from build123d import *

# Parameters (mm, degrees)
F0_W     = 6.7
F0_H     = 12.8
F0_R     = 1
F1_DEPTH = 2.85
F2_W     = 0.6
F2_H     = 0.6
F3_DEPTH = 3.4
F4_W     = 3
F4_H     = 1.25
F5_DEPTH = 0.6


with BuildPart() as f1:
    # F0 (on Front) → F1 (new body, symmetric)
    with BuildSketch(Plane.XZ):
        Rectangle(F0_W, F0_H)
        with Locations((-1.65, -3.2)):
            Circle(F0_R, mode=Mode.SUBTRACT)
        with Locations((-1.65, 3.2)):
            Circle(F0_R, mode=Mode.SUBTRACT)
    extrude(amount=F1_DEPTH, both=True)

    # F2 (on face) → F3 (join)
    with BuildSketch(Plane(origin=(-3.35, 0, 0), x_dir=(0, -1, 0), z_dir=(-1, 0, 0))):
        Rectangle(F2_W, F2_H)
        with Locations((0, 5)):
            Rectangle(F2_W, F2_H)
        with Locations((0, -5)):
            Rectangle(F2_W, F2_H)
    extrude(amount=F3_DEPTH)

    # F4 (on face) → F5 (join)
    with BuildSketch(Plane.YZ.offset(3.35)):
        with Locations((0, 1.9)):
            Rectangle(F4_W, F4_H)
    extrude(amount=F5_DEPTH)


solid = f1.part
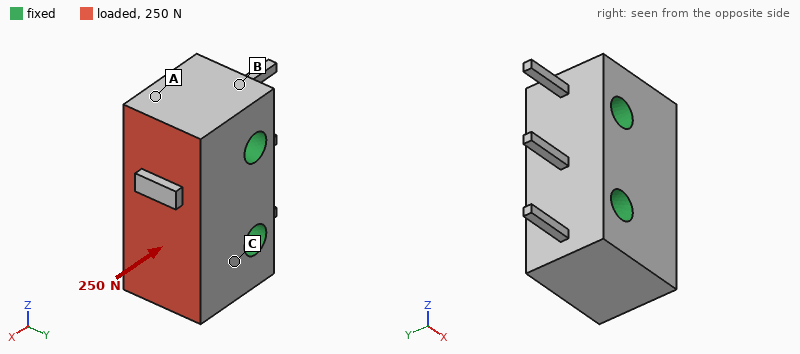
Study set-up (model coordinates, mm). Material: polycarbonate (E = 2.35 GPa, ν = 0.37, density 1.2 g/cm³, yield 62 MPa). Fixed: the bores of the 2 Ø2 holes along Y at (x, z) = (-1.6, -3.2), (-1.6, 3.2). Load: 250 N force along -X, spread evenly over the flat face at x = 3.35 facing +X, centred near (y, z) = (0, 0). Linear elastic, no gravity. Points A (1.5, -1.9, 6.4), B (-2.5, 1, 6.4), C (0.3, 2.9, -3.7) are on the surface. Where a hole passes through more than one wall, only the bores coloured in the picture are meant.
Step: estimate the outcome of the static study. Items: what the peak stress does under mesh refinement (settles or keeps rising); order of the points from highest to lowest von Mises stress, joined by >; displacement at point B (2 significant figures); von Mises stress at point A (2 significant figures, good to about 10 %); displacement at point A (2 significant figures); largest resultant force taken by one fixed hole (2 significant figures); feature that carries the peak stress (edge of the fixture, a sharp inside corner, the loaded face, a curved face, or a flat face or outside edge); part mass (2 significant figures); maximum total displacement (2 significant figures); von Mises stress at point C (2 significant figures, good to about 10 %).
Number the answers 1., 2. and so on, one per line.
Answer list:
1. keeps rising
2. C > A > B
3. 5.3 µm
4. 3.0 MPa
5. 8.8 µm
6. 130 N
7. edge of the fixture
8. 0.55 g
9. 12 µm
10. 5.1 MPa
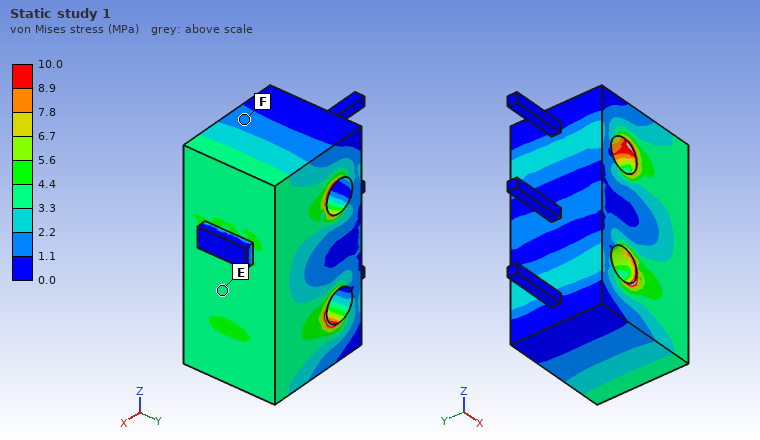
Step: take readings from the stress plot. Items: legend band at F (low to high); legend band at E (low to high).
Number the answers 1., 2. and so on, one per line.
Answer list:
1. 1.1 to 2.2 MPa
2. 3.3 to 4.4 MPa
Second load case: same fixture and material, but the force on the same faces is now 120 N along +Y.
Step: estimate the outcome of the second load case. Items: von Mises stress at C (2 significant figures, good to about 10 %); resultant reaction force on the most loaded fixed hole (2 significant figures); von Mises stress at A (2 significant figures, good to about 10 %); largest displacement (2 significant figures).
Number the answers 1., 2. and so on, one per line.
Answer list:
1. 8.0 MPa
2. 61 N
3. 2.0 MPa
4. 26 µm
